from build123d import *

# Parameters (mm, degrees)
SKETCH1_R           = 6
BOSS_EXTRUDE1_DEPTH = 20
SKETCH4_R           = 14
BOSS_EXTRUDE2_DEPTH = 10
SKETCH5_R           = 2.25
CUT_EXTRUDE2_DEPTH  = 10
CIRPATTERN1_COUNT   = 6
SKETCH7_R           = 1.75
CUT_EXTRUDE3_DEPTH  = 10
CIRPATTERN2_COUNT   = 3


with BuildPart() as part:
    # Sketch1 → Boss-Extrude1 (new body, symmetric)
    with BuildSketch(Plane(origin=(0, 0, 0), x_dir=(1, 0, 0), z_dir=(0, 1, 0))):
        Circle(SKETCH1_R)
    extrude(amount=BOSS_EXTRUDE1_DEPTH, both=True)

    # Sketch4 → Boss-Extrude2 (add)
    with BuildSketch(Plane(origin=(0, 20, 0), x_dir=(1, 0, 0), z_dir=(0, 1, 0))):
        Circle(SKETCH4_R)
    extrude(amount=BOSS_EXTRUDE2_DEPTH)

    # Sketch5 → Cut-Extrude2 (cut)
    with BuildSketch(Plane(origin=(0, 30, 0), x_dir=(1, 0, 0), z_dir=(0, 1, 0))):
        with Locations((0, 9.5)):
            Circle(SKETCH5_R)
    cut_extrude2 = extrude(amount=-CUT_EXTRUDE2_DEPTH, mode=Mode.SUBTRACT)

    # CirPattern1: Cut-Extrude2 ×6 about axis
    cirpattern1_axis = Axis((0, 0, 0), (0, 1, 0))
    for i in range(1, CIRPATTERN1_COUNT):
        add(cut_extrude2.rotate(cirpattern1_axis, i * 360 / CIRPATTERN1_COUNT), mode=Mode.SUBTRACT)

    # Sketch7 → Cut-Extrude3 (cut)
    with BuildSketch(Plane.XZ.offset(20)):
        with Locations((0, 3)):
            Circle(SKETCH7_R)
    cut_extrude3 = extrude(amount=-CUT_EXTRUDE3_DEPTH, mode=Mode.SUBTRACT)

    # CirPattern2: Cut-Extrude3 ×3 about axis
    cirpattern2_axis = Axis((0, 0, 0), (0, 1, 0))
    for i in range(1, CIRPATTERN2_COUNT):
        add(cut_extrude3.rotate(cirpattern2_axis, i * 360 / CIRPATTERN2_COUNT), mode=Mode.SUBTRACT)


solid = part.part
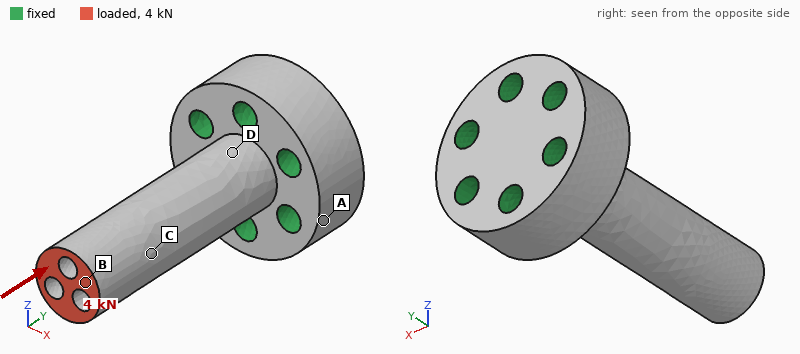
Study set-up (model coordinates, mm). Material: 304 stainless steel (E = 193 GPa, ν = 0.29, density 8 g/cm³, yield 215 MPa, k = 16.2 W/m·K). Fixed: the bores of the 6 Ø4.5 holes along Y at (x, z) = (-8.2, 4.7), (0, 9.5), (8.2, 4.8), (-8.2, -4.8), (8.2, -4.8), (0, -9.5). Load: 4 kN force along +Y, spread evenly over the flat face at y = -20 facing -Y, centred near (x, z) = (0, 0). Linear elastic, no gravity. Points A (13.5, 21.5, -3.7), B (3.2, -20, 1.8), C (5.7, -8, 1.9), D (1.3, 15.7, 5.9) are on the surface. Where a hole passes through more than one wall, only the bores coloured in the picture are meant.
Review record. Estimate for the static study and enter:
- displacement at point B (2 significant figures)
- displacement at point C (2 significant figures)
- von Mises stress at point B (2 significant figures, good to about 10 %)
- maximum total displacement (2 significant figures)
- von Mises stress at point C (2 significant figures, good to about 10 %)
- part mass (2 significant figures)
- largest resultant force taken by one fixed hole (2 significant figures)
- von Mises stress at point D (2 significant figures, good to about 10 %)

8.8 µm
6.0 µm
48 MPa
8.8 µm
42 MPa
76 g
760 N
34 MPa
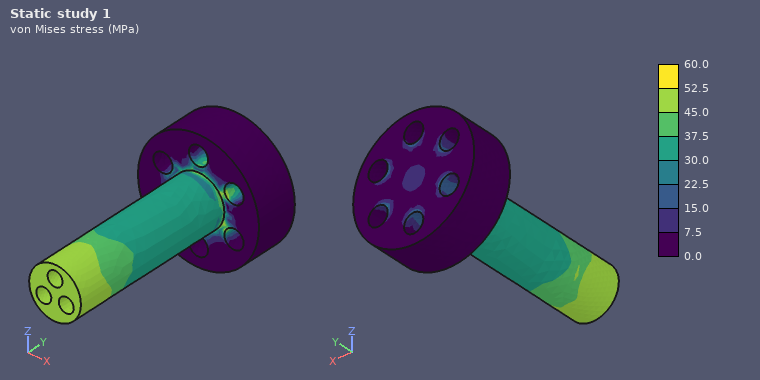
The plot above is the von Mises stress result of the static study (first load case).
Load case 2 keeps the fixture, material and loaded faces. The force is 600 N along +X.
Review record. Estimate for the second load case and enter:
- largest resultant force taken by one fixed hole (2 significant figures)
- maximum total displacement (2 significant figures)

960 N
82 µm
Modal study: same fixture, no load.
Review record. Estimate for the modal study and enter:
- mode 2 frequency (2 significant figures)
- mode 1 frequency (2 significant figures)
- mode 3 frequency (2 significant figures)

4900 Hz
4900 Hz
19 kHz
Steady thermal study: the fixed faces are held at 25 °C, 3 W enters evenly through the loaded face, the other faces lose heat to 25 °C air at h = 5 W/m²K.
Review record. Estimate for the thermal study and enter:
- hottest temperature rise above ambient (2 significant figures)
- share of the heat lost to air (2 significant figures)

70 K
12 %
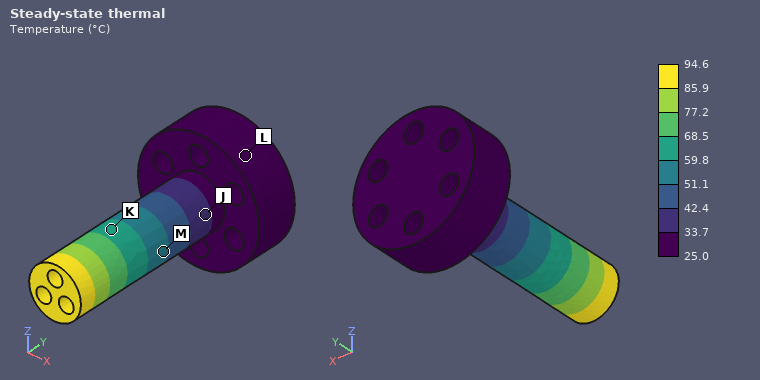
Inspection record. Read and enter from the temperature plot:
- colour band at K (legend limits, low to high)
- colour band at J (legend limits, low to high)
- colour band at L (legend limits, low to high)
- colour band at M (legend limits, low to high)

59.8 to 68.5 °C
33.7 to 42.4 °C
25.0 to 33.7 °C
51.1 to 59.8 °C
